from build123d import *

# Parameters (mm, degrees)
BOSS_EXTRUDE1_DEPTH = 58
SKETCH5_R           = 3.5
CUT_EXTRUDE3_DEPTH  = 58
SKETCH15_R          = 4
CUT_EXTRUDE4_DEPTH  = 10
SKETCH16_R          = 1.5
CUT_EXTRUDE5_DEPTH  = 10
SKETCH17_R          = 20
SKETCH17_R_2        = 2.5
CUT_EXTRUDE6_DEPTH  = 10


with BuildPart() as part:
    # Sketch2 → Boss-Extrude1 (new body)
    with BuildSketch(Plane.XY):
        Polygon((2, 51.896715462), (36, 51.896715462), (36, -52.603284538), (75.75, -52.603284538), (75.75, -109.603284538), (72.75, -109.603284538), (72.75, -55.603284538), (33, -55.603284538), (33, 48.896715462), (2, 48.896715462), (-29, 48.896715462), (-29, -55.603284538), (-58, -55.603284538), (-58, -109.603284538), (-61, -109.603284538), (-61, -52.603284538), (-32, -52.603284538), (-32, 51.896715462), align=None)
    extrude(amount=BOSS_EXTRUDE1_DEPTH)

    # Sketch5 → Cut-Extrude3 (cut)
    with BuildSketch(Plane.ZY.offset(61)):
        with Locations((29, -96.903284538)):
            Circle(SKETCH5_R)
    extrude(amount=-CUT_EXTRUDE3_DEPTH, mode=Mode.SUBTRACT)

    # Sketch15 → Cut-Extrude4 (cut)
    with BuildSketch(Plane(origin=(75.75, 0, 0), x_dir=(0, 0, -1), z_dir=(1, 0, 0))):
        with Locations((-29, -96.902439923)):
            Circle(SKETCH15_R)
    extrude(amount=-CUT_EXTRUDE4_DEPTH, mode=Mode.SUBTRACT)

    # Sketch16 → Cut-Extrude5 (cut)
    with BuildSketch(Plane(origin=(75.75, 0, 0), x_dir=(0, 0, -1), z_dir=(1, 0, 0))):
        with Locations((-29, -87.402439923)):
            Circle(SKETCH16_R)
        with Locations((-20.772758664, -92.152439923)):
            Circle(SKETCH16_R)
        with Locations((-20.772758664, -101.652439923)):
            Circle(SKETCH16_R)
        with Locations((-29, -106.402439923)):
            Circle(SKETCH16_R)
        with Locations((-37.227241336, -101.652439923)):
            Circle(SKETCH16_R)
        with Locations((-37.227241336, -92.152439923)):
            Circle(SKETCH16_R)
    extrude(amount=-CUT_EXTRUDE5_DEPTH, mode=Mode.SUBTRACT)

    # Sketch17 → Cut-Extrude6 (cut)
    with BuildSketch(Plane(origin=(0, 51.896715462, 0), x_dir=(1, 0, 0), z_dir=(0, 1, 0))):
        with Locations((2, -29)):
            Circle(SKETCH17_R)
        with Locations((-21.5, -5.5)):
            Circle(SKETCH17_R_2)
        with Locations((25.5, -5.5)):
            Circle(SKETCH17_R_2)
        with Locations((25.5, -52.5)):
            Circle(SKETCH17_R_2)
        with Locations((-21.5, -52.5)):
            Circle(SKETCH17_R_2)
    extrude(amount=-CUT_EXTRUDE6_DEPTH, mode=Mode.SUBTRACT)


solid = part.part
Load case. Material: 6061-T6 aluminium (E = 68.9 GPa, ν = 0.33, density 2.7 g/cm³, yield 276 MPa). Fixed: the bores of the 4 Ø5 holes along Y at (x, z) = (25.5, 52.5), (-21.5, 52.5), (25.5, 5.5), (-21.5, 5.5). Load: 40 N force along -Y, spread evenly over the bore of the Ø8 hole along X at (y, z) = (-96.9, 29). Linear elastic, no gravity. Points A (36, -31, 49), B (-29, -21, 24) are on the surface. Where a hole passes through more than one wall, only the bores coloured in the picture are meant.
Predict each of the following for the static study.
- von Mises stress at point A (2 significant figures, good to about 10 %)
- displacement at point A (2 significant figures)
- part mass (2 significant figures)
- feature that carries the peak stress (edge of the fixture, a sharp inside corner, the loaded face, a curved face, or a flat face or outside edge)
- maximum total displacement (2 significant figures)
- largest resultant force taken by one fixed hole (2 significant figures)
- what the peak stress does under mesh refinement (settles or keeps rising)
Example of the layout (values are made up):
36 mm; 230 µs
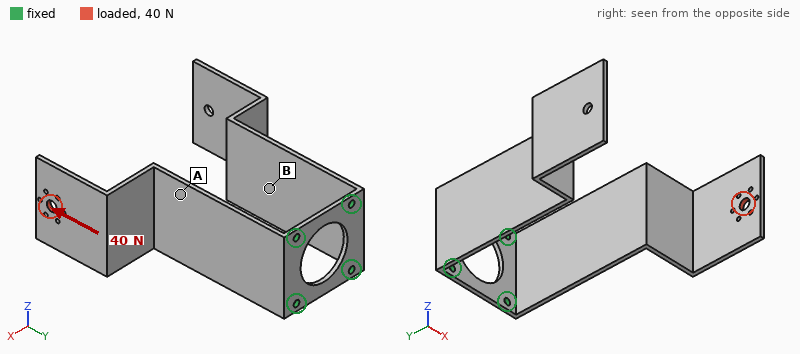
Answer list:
18 MPa; 0.71 mm; 200 g; edge of the fixture; 2.5 mm; 22 N; keeps rising
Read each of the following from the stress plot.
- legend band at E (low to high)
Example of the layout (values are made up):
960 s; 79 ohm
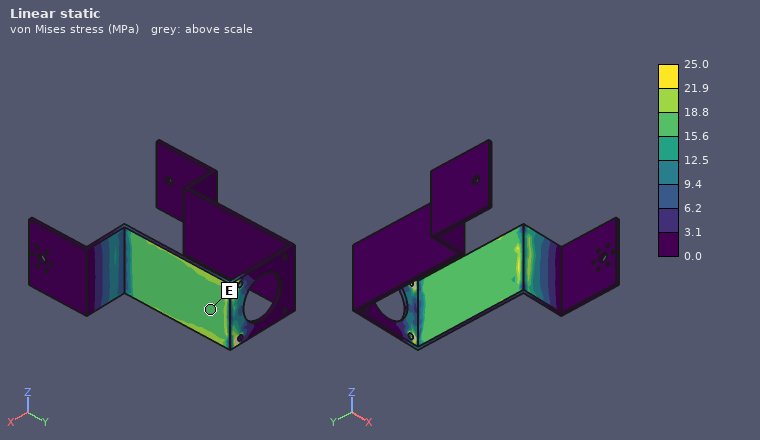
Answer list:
15.6 to 18.8 MPa
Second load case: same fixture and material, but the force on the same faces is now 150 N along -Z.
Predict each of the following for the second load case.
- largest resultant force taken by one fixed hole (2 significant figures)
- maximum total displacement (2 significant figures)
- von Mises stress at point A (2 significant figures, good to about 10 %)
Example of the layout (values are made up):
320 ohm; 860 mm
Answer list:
510 N; 2.2 mm; 51 MPa
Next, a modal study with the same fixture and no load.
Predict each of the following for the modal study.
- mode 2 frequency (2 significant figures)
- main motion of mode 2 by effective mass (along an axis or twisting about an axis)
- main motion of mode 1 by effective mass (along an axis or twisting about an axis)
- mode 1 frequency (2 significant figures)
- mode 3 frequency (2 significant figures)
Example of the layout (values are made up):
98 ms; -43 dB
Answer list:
77 Hz; along X; along X; 73 Hz; 240 Hz
